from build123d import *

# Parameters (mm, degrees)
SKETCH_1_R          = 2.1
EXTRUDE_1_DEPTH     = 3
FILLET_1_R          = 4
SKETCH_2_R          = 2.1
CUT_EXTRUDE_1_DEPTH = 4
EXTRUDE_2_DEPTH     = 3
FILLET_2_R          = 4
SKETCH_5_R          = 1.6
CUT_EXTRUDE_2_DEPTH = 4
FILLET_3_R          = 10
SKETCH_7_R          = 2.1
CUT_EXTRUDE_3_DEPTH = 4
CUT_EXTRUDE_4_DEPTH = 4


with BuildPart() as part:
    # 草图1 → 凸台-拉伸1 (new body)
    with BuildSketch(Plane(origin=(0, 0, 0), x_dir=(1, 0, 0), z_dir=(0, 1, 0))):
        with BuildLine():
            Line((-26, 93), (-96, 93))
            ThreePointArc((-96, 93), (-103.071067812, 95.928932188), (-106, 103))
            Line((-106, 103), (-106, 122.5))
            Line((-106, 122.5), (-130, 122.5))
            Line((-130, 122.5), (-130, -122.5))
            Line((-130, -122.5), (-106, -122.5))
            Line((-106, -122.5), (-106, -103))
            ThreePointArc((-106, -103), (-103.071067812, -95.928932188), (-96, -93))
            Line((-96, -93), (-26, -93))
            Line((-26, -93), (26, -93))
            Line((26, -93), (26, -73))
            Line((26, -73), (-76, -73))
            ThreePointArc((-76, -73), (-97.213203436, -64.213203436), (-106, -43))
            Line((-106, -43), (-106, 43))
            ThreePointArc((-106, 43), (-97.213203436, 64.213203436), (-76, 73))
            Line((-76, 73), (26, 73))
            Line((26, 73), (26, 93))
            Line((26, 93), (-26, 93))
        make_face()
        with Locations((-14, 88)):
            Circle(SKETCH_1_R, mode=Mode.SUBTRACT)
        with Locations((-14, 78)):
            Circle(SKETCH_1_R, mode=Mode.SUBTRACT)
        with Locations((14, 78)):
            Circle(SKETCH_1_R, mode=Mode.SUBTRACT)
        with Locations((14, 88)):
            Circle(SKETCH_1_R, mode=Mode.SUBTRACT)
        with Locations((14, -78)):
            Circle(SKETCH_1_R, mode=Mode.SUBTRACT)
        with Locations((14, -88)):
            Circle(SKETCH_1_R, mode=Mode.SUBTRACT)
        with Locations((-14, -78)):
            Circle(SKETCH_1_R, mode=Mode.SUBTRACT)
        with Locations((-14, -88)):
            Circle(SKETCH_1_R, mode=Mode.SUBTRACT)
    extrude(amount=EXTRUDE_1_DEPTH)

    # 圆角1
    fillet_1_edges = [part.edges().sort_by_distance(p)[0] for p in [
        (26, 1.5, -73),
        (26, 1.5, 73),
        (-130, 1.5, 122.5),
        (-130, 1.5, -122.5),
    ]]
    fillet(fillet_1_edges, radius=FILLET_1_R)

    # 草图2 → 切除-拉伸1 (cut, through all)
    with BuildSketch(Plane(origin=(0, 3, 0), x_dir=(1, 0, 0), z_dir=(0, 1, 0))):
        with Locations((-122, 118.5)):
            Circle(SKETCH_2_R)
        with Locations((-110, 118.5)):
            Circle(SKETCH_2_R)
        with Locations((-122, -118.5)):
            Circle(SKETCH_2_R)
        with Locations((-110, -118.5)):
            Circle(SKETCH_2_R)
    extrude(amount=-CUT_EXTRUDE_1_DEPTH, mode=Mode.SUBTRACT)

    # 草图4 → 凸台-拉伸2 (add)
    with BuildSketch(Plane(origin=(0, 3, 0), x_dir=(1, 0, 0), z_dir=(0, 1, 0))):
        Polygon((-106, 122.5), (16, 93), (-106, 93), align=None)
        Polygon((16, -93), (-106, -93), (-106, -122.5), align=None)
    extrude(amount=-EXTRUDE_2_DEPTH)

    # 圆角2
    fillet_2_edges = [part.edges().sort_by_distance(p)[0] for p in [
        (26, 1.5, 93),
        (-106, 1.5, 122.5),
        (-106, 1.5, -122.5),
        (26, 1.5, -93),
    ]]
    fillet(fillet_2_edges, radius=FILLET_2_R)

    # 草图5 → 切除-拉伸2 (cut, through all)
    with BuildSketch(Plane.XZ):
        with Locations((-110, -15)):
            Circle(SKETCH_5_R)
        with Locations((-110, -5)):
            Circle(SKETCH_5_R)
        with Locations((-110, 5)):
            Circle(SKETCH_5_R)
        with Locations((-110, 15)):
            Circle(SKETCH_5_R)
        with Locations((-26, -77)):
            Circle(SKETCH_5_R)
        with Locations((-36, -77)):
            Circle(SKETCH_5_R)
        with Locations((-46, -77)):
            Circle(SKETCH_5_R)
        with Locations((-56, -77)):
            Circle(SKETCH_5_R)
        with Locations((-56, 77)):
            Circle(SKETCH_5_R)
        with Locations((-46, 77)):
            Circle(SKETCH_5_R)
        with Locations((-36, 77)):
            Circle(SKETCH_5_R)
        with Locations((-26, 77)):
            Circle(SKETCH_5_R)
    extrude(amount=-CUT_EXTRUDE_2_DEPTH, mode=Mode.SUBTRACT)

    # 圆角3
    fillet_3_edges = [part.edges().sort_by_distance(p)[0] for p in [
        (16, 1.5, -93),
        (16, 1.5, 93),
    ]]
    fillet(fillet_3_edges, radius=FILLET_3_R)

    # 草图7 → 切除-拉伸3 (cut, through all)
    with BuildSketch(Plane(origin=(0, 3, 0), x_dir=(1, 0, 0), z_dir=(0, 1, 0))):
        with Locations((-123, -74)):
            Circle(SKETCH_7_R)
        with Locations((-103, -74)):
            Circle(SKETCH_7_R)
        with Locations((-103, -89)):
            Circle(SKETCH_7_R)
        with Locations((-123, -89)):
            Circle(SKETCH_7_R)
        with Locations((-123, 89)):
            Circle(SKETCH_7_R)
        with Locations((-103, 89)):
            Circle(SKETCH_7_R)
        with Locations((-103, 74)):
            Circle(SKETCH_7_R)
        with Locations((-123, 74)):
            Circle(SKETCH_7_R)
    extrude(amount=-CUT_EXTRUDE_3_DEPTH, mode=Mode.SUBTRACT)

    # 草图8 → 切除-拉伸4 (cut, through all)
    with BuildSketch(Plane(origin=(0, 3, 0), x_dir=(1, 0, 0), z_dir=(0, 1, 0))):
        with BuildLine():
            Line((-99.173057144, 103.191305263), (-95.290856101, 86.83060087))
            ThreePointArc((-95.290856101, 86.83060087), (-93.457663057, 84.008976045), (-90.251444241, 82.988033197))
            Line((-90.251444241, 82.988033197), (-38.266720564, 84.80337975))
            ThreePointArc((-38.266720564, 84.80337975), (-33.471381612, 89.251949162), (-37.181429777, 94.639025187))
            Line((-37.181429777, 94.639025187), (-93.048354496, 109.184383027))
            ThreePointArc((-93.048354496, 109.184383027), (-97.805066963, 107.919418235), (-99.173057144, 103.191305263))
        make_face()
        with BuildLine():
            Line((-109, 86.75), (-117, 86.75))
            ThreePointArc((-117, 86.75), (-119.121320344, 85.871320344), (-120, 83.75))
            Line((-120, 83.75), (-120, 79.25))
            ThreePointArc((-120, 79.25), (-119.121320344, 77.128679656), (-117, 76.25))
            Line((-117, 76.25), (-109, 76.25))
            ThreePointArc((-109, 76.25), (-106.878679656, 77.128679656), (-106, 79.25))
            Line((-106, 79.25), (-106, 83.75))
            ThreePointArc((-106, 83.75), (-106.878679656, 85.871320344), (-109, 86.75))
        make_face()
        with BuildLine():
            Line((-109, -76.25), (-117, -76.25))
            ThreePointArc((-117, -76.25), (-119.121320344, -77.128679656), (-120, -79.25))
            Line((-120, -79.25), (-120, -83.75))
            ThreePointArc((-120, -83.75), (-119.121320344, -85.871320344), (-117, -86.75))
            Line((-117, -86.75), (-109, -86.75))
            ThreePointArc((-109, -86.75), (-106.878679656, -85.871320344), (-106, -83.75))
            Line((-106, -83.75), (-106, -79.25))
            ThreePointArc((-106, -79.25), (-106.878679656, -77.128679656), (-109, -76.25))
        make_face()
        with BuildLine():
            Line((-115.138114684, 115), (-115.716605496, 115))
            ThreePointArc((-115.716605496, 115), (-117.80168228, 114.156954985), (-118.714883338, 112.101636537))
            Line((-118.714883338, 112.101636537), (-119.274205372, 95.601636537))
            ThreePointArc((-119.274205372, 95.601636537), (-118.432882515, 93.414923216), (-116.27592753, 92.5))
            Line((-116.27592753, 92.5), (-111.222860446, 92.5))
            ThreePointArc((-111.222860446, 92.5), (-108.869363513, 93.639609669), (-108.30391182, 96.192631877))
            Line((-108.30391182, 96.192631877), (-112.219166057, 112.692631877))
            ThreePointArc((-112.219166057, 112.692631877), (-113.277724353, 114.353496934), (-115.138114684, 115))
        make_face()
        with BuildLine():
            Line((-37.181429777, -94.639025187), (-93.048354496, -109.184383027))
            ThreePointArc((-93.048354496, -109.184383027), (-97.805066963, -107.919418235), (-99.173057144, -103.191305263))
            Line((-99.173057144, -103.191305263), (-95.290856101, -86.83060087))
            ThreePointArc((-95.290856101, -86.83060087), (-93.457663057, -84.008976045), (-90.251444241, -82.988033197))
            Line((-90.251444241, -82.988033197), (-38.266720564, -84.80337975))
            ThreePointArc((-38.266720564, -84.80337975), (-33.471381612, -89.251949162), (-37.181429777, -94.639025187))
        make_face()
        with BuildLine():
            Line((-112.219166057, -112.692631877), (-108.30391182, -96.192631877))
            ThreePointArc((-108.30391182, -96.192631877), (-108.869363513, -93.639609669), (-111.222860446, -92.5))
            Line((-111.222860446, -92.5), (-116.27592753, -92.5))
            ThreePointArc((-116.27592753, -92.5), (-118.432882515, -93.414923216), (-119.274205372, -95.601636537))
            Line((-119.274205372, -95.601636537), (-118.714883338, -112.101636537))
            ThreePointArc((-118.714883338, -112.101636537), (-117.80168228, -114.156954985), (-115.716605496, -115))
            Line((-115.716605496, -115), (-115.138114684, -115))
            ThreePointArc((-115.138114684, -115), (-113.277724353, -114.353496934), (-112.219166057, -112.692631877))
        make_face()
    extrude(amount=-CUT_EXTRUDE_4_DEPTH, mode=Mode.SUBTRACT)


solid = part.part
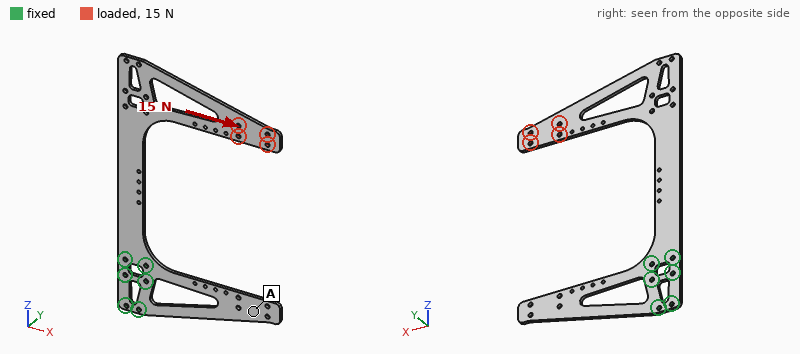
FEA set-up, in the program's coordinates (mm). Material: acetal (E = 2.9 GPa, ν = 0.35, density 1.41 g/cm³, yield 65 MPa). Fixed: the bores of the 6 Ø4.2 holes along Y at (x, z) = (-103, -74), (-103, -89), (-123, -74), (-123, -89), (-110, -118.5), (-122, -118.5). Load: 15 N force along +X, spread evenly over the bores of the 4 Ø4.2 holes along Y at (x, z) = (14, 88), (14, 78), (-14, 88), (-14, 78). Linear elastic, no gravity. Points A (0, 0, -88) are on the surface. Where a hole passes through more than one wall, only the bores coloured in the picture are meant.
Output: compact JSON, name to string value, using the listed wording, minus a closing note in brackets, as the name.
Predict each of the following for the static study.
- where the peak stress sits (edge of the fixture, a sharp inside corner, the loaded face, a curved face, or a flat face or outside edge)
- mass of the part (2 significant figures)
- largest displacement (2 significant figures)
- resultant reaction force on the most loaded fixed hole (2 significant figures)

{"where the peak stress sits": "a curved face", "mass of the part": "50 g", "largest displacement": "3.0 mm", "resultant reaction force on the most loaded fixed hole": "94 N"}
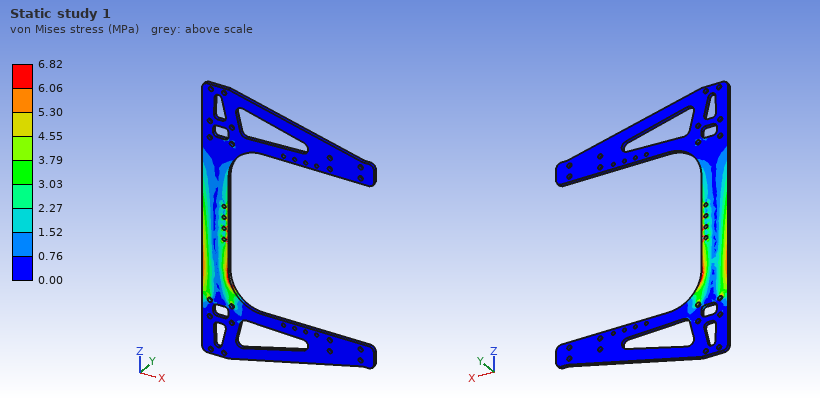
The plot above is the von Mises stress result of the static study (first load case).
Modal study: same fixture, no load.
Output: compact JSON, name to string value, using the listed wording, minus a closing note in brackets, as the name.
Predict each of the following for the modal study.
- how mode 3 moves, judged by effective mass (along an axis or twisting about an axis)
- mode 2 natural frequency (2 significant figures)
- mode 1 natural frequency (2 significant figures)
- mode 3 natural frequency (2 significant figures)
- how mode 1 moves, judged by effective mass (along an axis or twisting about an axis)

{"how mode 3 moves, judged by effective mass": "along Y", "mode 2 natural frequency": "27 Hz", "mode 1 natural frequency": "11 Hz", "mode 3 natural frequency": "43 Hz", "how mode 1 moves, judged by effective mass": "along Y"}
